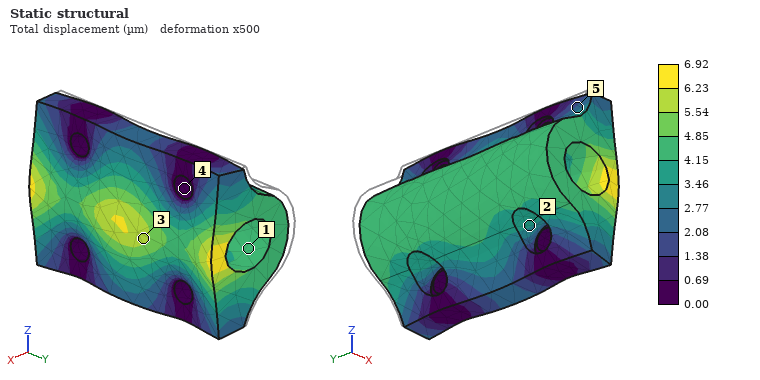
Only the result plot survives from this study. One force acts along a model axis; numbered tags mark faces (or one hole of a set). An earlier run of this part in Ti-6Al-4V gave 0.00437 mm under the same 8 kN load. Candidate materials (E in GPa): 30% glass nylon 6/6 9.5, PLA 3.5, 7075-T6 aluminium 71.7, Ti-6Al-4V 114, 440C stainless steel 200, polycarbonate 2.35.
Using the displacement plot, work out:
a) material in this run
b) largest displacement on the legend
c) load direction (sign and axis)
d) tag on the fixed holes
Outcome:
7075-T6 aluminium
6.92 µm
+X
4
